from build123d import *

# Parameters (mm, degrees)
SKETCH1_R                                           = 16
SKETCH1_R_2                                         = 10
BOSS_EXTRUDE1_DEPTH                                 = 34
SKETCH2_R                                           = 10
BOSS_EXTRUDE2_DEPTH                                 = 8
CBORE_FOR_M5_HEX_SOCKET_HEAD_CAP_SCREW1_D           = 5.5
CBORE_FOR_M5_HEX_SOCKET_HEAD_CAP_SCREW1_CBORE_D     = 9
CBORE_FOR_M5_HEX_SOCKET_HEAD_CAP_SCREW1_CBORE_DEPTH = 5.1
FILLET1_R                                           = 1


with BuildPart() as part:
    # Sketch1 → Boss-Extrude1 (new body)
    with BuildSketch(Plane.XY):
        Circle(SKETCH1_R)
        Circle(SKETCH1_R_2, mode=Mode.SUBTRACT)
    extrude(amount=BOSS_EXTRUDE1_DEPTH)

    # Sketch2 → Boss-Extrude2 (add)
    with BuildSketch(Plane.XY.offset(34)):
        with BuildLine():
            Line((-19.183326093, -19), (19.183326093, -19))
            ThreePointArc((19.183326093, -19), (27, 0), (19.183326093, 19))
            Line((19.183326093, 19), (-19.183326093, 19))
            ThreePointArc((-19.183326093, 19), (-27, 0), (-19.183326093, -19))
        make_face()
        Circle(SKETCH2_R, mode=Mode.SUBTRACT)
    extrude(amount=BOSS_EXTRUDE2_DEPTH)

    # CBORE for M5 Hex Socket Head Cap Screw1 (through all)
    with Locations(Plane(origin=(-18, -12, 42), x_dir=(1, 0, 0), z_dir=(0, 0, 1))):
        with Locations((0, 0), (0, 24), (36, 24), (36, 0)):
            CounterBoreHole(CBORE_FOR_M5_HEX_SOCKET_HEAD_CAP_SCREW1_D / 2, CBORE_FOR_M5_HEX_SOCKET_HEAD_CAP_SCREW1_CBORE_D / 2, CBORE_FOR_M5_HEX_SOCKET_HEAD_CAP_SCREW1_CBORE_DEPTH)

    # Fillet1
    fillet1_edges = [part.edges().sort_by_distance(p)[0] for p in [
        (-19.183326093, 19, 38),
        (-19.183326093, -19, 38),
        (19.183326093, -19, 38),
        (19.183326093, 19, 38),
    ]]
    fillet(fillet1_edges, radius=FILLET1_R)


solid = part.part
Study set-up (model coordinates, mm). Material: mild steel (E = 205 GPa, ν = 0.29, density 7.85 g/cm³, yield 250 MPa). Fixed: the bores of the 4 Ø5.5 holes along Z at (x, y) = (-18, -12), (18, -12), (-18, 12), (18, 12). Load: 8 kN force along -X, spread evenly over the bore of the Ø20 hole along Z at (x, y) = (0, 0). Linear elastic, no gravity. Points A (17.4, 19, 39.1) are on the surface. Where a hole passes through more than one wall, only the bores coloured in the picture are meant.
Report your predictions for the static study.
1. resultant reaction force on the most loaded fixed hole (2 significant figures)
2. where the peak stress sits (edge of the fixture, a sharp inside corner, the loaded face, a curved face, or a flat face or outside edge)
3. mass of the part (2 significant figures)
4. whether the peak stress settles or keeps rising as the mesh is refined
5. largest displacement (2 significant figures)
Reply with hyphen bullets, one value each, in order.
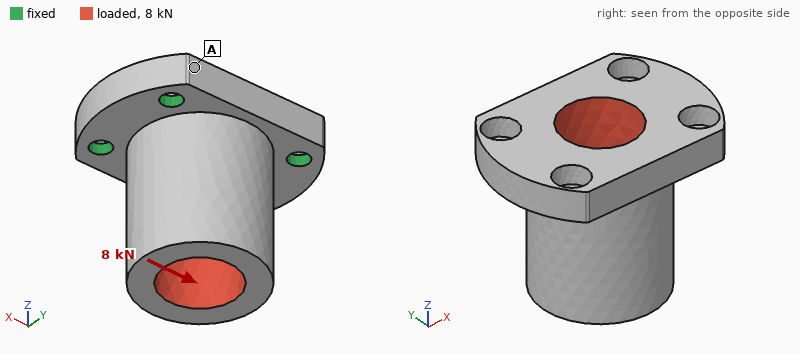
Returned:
- 2.7 kN
- edge of the fixture
- 220 g
- keeps rising
- 21 µm
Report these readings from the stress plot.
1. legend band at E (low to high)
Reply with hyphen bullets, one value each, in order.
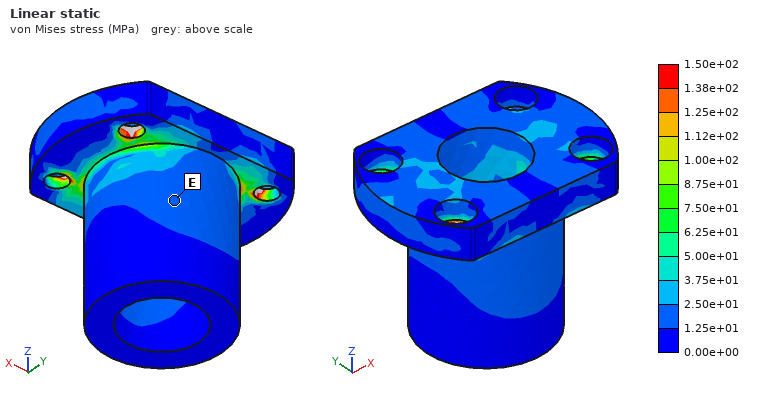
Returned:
- 1.25e+01 to 2.50e+01 MPa
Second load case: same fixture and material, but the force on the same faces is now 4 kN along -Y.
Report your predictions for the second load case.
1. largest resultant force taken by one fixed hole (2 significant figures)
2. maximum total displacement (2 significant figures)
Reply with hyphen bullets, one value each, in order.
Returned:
- 1.6 kN
- 17 µm
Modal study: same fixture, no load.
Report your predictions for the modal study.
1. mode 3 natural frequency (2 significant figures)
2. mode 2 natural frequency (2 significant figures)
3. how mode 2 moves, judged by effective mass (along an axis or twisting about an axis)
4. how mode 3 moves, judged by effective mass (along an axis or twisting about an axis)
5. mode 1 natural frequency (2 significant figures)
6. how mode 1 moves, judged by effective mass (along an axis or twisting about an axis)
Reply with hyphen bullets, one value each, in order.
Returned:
- 14 kHz
- 9100 Hz
- along X
- along Z
- 7000 Hz
- along Y
